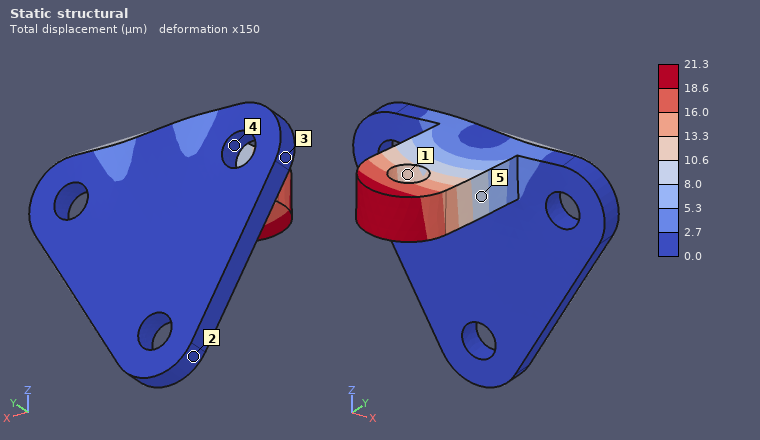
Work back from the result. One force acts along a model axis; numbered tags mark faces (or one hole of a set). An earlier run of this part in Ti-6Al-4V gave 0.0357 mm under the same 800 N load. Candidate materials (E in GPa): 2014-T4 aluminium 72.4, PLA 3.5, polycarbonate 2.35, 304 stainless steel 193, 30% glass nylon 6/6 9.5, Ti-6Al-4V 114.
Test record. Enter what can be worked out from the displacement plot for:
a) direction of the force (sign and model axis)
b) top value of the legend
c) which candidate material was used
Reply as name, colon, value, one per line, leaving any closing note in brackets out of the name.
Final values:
direction of the force: -X
top value of the legend: 21.3 µm
which candidate material was used: 304 stainless steel
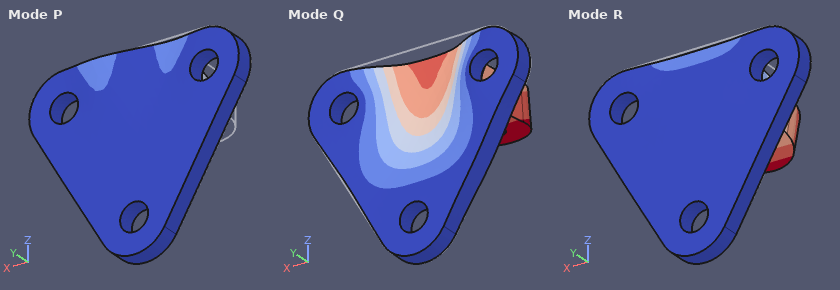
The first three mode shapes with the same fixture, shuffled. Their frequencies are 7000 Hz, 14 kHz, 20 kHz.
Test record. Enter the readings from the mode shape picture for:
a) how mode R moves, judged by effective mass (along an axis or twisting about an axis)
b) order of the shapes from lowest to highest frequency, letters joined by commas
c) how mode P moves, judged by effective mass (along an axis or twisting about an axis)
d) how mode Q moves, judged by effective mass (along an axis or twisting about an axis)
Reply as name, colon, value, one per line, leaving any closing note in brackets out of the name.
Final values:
how mode R moves, judged by effective mass: along Z
order of the shapes from lowest to highest frequency, letters joined by commas: R, P, Q
how mode P moves, judged by effective mass: along X
how mode Q moves, judged by effective mass: along Y
